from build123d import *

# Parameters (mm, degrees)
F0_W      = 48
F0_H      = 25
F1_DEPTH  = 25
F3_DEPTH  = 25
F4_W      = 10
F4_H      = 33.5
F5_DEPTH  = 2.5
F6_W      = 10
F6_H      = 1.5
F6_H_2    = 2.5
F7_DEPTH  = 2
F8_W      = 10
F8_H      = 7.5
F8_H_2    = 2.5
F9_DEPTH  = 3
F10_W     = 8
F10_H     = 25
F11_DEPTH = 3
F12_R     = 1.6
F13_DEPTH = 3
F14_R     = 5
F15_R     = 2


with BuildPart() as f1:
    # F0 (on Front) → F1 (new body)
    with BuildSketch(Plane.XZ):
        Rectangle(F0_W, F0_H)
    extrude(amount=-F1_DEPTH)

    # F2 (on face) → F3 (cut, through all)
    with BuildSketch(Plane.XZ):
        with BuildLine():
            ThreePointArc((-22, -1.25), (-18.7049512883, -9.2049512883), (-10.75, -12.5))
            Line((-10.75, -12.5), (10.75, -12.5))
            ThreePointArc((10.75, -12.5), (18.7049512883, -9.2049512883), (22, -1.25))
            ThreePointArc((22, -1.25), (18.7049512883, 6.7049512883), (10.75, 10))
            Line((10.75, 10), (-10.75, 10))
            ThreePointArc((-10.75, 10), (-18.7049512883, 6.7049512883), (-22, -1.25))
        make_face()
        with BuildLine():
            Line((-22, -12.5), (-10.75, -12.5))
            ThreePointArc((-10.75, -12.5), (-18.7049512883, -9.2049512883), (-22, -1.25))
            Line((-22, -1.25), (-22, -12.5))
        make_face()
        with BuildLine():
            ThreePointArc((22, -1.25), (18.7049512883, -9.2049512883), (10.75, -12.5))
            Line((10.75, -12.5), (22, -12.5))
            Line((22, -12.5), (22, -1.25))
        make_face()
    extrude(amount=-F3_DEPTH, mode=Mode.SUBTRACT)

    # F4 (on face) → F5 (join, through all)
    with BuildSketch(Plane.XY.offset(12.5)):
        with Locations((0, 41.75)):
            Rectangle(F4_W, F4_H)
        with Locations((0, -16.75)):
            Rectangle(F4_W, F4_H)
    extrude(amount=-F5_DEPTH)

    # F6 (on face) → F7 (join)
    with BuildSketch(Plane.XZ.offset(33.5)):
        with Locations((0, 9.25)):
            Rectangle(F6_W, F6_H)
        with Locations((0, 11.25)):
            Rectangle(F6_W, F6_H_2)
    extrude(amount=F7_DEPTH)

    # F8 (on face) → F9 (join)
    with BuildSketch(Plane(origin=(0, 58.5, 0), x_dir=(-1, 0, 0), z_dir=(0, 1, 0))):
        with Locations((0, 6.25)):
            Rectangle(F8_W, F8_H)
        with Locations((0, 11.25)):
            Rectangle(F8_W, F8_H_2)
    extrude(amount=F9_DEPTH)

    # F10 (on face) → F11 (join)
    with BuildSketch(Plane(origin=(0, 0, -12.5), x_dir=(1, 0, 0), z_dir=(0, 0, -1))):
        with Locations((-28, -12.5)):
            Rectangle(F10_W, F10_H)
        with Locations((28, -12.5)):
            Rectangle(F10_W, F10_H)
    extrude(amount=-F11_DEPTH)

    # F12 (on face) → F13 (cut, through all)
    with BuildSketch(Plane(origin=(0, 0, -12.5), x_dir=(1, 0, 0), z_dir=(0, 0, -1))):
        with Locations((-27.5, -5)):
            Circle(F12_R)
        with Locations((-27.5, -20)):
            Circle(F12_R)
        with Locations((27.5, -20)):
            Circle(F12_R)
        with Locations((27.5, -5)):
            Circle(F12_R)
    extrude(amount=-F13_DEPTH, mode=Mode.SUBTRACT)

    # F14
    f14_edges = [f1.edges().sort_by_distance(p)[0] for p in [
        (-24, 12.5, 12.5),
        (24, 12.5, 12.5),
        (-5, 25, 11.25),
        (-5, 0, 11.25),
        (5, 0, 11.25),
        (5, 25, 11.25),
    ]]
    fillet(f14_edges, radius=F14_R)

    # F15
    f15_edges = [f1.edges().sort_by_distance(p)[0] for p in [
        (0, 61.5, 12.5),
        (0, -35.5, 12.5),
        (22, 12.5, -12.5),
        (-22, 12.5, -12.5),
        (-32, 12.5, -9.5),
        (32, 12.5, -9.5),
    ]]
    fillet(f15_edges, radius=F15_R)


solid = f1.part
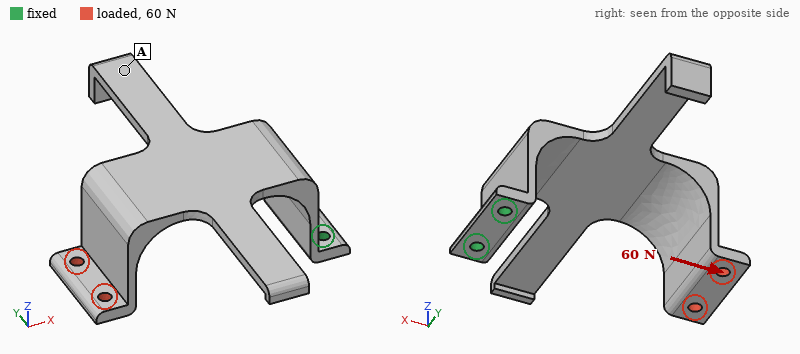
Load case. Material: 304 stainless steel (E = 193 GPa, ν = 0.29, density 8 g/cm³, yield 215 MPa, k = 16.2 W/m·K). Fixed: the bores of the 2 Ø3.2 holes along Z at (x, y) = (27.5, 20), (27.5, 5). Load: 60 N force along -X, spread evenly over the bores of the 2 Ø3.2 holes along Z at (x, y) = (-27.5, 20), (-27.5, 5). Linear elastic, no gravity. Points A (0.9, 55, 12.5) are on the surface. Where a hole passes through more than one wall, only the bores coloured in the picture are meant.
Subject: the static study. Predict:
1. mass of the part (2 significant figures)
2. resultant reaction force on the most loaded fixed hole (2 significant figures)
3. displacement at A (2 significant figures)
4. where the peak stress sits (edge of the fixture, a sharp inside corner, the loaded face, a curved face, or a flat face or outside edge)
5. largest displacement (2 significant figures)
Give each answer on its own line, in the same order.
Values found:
76 g
30 N
0.053 mm
a curved face
0.34 mm
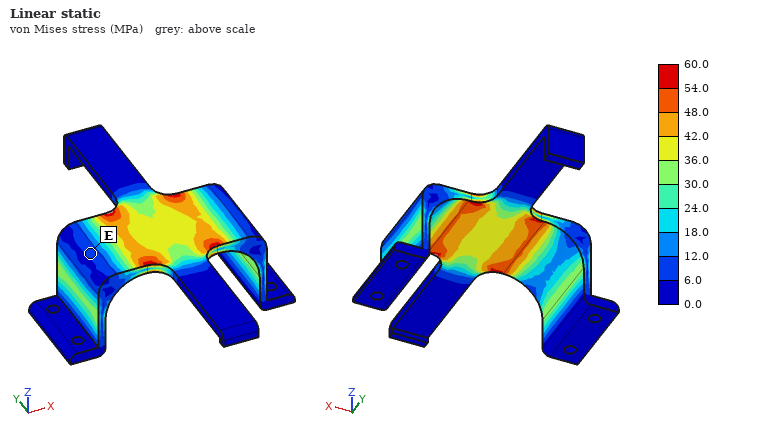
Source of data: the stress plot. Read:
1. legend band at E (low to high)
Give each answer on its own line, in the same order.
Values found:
6.0 to 12.0 MPa
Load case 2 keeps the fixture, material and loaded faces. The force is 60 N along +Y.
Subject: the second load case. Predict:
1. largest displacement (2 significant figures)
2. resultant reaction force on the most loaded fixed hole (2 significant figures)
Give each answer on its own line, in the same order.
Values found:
0.31 mm
190 N
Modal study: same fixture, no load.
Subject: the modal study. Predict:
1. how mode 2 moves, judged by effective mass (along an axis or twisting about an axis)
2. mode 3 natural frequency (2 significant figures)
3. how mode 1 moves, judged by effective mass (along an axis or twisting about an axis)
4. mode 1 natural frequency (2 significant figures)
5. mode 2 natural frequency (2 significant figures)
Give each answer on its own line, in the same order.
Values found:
along Y
780 Hz
along Z
260 Hz
480 Hz
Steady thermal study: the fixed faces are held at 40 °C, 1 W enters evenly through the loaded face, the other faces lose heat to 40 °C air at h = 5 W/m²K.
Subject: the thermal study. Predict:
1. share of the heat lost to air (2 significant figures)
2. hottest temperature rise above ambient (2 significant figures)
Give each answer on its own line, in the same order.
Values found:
65 %
47 K
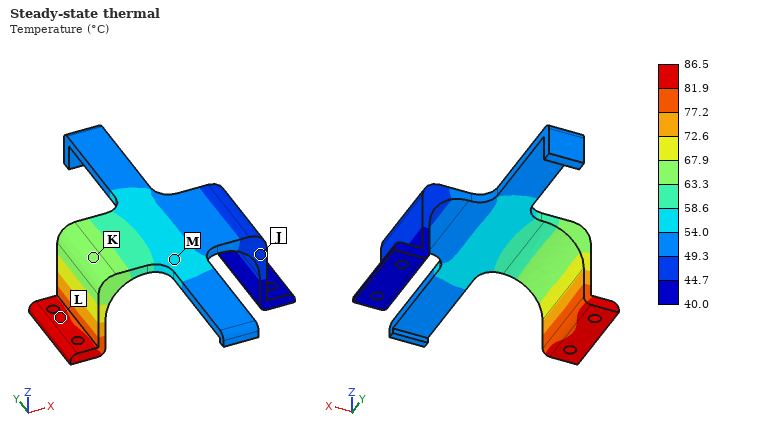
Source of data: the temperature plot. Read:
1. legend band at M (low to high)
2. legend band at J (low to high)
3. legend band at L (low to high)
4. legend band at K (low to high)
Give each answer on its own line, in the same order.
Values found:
54.0 to 58.6 °C
44.7 to 49.3 °C
81.9 to 86.5 °C
63.3 to 67.9 °C
